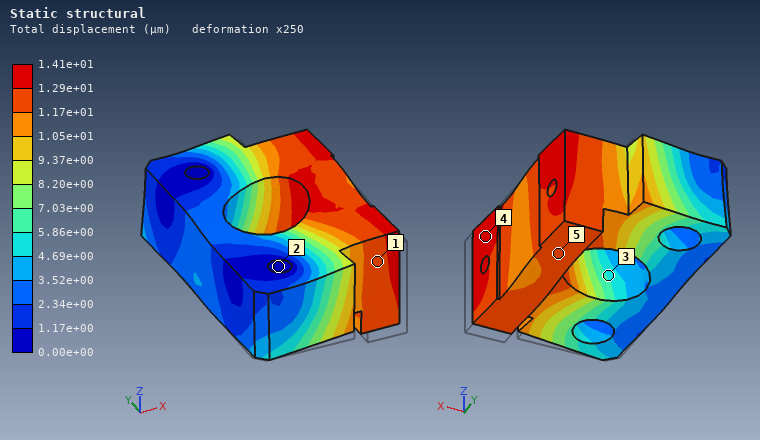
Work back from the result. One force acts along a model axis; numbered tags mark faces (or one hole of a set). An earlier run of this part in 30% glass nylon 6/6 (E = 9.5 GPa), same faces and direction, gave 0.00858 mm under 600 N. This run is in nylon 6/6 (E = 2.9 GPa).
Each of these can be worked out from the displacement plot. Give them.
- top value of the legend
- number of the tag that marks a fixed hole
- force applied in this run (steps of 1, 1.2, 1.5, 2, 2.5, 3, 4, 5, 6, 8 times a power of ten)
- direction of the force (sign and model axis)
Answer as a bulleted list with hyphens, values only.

- 1.41e+01 µm
- 2
- 300 N
- +Y
